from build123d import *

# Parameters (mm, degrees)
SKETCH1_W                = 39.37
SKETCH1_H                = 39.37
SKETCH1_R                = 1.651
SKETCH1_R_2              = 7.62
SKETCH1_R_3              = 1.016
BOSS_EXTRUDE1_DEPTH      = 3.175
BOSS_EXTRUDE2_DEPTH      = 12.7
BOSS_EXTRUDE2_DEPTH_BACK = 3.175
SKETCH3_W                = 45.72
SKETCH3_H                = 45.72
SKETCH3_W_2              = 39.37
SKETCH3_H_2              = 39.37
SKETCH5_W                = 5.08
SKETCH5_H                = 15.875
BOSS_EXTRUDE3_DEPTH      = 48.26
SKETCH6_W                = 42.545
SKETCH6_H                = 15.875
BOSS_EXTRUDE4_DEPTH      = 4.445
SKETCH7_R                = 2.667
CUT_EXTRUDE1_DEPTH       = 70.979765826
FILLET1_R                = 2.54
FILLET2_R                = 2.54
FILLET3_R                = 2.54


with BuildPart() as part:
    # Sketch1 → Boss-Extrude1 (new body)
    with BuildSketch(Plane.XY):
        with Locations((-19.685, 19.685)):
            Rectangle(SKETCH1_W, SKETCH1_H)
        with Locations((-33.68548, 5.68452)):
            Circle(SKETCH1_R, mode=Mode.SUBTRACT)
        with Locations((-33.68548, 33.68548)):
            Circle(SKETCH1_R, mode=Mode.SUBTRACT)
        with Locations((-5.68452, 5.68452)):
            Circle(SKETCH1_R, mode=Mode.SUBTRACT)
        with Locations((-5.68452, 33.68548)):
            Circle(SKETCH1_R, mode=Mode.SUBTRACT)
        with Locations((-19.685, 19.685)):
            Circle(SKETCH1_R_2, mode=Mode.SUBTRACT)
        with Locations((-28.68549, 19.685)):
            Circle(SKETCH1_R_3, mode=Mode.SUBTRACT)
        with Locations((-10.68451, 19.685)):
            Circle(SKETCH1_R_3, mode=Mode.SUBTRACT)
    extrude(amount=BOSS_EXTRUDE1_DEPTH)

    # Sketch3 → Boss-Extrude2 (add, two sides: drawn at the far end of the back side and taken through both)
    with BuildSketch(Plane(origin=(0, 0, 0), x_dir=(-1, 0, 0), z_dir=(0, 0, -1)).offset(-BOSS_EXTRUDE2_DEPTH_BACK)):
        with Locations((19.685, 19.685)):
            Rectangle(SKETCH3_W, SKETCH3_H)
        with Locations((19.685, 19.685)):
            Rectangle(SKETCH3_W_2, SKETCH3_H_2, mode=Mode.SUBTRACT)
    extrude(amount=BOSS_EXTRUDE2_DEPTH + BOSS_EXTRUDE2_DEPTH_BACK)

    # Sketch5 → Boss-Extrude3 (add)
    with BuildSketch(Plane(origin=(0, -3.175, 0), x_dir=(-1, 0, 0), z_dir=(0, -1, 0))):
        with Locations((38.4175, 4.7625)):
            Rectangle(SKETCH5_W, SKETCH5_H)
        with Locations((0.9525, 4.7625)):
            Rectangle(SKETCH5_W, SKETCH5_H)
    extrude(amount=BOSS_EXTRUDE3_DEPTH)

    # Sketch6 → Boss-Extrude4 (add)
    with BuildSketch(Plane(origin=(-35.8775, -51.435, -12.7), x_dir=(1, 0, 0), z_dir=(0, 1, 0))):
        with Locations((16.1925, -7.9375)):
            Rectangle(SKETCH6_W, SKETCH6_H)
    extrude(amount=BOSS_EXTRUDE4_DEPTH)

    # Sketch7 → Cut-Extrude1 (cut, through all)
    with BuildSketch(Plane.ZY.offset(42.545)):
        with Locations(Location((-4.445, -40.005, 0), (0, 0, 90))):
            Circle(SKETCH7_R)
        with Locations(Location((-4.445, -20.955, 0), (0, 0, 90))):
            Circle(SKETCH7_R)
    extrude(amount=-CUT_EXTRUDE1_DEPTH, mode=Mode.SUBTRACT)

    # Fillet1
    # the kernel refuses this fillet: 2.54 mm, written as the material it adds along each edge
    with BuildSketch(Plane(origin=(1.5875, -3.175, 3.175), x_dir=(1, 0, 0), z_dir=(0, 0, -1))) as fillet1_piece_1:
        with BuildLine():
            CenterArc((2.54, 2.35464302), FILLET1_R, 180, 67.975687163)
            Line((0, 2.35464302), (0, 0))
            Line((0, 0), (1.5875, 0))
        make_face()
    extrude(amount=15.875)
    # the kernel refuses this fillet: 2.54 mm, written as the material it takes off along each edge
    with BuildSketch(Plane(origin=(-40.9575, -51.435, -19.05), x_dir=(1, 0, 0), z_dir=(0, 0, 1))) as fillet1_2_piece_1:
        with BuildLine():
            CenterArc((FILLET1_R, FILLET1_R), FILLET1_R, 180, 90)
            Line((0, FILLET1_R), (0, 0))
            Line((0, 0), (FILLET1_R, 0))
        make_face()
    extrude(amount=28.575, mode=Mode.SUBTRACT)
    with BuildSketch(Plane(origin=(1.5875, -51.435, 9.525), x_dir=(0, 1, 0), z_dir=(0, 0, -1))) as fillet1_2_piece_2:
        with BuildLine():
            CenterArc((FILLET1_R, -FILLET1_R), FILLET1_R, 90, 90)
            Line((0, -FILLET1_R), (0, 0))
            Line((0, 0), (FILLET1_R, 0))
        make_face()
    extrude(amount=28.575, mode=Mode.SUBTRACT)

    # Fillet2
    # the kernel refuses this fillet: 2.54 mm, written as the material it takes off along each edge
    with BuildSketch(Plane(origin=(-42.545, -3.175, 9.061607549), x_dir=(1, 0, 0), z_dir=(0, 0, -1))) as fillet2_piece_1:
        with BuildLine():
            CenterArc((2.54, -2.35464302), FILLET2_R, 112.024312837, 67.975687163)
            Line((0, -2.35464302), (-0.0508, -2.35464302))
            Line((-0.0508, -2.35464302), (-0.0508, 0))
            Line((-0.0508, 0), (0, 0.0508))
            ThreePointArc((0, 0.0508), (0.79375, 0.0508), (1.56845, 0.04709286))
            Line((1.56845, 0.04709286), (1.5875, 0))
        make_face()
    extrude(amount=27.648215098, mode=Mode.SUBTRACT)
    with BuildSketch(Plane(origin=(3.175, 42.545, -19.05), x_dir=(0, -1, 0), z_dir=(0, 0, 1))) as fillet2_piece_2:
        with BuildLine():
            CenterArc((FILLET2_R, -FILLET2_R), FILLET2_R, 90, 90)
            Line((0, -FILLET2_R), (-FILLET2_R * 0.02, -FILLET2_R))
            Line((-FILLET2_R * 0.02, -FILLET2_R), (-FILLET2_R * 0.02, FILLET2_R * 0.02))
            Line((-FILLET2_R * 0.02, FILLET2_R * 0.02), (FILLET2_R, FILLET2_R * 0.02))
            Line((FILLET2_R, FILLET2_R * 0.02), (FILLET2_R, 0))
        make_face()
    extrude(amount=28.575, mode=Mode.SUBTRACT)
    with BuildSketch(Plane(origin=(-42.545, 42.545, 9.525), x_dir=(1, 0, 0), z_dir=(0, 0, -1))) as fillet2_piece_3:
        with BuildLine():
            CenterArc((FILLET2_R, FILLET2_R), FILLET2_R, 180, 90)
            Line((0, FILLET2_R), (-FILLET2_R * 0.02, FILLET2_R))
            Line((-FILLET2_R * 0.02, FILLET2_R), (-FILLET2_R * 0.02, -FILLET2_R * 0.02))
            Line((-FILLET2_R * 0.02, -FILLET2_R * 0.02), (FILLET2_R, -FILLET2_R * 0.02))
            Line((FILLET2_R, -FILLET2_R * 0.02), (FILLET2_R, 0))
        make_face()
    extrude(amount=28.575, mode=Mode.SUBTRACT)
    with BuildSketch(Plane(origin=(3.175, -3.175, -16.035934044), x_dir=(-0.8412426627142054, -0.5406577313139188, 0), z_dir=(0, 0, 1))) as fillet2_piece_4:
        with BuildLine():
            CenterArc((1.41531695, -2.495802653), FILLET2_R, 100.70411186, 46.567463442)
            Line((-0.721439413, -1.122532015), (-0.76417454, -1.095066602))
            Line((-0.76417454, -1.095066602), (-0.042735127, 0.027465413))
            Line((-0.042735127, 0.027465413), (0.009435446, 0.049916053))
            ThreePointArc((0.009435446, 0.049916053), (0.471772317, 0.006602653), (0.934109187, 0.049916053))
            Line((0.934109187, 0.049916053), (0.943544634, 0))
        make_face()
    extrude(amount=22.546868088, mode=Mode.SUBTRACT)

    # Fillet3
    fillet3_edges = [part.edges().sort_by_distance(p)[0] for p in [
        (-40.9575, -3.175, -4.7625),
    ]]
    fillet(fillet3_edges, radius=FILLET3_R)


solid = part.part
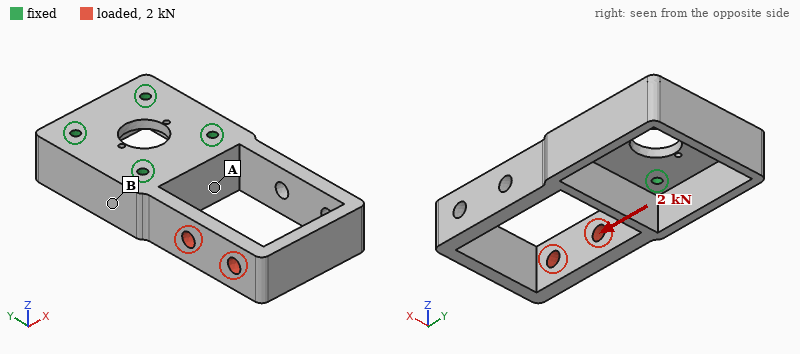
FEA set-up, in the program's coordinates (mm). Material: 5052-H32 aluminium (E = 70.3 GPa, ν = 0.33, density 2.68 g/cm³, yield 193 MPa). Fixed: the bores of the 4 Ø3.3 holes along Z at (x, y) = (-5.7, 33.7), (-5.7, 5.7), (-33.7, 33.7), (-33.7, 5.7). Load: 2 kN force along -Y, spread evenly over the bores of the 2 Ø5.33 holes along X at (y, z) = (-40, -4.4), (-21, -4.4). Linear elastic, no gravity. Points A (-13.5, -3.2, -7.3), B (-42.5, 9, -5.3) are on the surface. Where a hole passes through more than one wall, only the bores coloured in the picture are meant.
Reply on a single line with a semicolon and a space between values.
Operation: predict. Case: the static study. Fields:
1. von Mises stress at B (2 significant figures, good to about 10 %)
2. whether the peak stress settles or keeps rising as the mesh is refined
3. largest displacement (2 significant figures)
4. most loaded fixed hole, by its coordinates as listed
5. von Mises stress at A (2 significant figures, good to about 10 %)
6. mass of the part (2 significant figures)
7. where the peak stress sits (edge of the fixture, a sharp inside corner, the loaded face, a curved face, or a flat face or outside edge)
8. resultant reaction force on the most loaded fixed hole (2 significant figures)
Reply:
27 MPa; keeps rising; 81 µm; (-33.7, 5.7); 8.4 MPa; 60 g; edge of the fixture; 1.4 kN
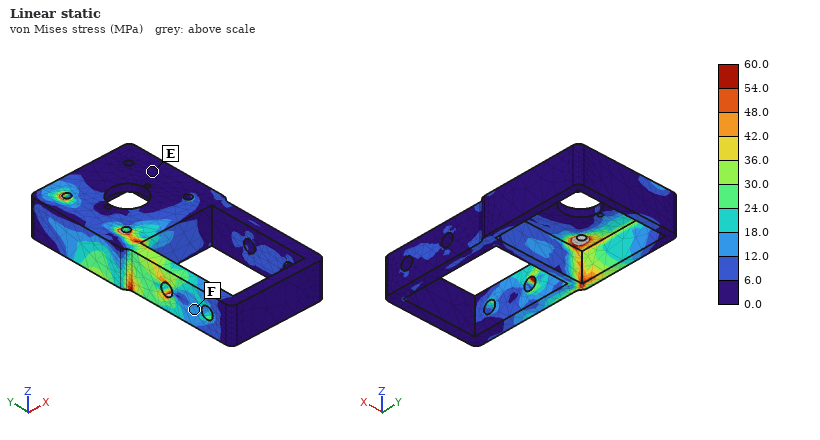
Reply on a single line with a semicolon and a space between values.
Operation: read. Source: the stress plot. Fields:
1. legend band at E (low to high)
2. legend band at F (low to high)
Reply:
0.0 to 6.0 MPa; 12.0 to 18.0 MPa
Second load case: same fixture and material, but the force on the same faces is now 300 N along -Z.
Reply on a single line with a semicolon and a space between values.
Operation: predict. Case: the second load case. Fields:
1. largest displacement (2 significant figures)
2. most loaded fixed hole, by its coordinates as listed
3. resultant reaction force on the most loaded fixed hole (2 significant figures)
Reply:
0.14 mm; (-33.7, 5.7); 650 N
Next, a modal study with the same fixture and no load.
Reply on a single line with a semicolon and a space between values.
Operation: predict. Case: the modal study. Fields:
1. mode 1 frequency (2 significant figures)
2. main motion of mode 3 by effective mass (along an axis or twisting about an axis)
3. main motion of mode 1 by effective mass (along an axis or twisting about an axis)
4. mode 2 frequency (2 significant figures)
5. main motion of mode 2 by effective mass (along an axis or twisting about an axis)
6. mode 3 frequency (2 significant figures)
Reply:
1700 Hz; twisting about Y; along X; 2000 Hz; along Z; 3100 Hz
